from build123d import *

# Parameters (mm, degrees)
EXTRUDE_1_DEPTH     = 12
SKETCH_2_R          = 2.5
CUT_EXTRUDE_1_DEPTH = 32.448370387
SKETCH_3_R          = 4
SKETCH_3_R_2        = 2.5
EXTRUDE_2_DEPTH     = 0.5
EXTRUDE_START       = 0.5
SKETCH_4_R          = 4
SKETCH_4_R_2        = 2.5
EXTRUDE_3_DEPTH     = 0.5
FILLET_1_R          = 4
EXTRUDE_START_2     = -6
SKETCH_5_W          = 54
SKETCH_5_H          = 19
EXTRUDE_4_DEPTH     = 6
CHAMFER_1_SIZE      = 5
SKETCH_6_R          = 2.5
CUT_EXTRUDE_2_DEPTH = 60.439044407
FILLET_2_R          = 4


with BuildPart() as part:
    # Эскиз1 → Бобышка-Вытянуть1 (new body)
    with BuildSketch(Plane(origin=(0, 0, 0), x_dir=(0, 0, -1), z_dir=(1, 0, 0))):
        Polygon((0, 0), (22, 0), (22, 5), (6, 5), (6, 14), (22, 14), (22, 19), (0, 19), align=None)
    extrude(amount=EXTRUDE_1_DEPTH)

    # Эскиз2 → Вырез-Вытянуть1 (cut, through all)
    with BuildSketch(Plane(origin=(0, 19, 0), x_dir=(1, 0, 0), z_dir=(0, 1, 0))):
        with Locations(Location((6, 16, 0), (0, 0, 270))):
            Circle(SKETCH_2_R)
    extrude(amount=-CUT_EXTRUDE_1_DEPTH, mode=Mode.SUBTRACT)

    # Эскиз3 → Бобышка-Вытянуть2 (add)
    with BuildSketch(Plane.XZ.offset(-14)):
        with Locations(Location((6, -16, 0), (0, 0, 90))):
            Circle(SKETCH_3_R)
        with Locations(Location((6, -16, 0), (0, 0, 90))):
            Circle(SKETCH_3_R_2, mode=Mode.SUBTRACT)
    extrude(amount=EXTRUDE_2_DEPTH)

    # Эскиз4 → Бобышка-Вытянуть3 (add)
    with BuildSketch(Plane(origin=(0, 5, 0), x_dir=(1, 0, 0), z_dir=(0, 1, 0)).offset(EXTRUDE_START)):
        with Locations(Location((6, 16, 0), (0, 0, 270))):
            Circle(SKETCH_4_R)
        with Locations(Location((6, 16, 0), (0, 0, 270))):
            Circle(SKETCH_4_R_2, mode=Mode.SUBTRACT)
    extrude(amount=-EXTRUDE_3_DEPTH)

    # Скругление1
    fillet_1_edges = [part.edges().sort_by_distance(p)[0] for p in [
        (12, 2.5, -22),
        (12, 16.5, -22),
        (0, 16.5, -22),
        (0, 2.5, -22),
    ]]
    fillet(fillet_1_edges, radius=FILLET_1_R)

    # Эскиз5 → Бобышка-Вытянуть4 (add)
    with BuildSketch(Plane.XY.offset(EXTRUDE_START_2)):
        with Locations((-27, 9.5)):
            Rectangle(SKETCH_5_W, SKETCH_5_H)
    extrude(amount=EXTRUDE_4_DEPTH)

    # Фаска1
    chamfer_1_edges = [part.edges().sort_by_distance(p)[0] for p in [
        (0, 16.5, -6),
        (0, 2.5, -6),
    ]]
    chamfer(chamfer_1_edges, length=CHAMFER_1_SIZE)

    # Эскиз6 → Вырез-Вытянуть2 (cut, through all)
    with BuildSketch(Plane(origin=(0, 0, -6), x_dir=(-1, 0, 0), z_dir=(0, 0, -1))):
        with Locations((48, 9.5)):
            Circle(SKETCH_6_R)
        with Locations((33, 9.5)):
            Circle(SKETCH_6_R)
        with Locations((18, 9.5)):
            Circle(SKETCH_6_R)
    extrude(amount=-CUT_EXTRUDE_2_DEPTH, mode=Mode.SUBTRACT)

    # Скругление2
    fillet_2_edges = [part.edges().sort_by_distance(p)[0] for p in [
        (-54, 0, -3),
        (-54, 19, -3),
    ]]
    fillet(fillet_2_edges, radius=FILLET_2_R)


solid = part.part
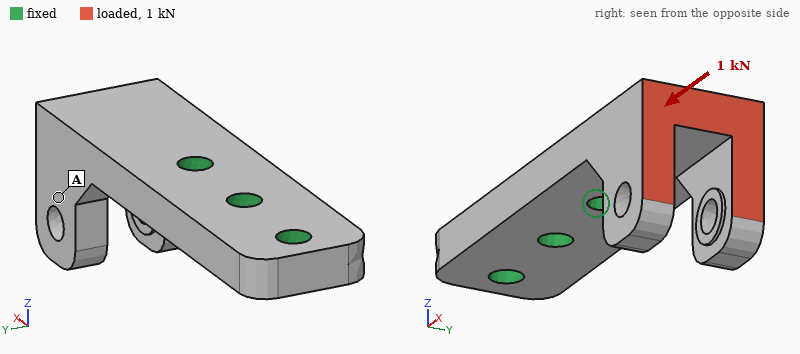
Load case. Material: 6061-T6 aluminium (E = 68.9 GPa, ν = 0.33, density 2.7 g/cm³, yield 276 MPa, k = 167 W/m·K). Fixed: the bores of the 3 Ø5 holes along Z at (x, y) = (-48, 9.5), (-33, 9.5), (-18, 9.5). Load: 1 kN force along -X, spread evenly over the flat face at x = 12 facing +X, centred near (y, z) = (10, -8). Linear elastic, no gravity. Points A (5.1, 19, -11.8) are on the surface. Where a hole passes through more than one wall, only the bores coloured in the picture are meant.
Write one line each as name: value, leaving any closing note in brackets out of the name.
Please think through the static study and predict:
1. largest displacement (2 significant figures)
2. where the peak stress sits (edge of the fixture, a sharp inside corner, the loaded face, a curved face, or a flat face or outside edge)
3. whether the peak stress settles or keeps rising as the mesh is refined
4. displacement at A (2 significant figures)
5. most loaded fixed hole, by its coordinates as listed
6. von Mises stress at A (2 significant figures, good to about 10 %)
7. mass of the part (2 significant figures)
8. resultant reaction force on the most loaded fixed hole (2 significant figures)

largest displacement: 90 µm
where the peak stress sits: edge of the fixture
whether the peak stress settles or keeps rising as the mesh is refined: keeps rising
displacement at A: 55 µm
most loaded fixed hole, by its coordinates as listed: (-18, 9.5)
von Mises stress at A: 10 MPa
mass of the part: 24 g
resultant reaction force on the most loaded fixed hole: 840 N
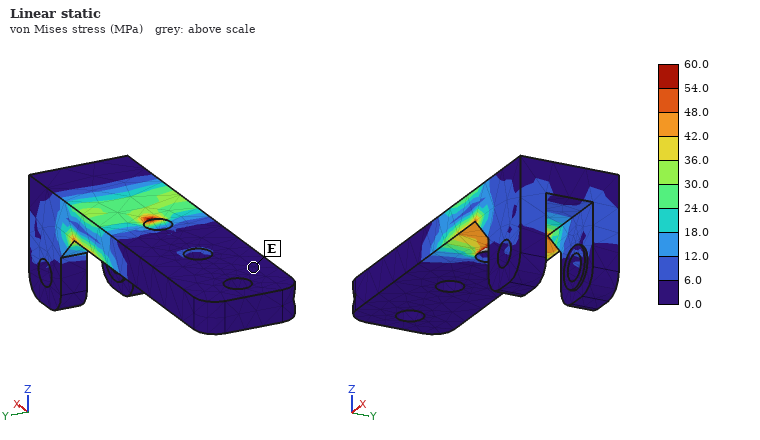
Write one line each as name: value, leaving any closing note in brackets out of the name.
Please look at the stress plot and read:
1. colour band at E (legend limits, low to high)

colour band at E: 0.0 to 6.0 MPa
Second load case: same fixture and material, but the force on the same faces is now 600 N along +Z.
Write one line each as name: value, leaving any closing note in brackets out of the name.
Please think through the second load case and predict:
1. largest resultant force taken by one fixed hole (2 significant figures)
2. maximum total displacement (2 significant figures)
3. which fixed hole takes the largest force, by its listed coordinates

largest resultant force taken by one fixed hole: 870 N
maximum total displacement: 0.25 mm
which fixed hole takes the largest force, by its listed coordinates: (-18, 9.5)
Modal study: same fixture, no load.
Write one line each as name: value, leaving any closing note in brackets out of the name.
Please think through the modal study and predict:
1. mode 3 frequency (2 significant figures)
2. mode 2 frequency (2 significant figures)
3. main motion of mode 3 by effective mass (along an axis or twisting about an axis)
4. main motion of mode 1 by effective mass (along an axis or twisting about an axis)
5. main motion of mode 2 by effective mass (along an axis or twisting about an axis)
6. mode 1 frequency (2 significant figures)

mode 3 frequency: 9300 Hz
mode 2 frequency: 5500 Hz
main motion of mode 3 by effective mass: along Y
main motion of mode 1 by effective mass: along Z
main motion of mode 2 by effective mass: along Y
mode 1 frequency: 3500 Hz
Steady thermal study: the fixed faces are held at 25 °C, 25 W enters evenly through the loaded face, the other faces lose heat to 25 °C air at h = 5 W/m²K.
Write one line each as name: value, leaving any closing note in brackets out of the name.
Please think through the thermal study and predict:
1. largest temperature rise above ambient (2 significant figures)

largest temperature rise above ambient: 34 K
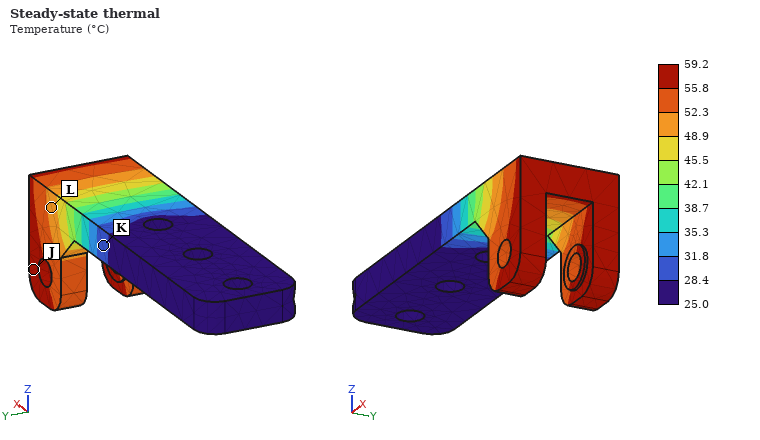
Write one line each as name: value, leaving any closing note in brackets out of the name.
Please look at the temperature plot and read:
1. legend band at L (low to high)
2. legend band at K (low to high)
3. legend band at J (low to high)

legend band at L: 48.9 to 52.3 °C
legend band at K: 28.4 to 31.8 °C
legend band at J: 55.8 to 59.2 °C
